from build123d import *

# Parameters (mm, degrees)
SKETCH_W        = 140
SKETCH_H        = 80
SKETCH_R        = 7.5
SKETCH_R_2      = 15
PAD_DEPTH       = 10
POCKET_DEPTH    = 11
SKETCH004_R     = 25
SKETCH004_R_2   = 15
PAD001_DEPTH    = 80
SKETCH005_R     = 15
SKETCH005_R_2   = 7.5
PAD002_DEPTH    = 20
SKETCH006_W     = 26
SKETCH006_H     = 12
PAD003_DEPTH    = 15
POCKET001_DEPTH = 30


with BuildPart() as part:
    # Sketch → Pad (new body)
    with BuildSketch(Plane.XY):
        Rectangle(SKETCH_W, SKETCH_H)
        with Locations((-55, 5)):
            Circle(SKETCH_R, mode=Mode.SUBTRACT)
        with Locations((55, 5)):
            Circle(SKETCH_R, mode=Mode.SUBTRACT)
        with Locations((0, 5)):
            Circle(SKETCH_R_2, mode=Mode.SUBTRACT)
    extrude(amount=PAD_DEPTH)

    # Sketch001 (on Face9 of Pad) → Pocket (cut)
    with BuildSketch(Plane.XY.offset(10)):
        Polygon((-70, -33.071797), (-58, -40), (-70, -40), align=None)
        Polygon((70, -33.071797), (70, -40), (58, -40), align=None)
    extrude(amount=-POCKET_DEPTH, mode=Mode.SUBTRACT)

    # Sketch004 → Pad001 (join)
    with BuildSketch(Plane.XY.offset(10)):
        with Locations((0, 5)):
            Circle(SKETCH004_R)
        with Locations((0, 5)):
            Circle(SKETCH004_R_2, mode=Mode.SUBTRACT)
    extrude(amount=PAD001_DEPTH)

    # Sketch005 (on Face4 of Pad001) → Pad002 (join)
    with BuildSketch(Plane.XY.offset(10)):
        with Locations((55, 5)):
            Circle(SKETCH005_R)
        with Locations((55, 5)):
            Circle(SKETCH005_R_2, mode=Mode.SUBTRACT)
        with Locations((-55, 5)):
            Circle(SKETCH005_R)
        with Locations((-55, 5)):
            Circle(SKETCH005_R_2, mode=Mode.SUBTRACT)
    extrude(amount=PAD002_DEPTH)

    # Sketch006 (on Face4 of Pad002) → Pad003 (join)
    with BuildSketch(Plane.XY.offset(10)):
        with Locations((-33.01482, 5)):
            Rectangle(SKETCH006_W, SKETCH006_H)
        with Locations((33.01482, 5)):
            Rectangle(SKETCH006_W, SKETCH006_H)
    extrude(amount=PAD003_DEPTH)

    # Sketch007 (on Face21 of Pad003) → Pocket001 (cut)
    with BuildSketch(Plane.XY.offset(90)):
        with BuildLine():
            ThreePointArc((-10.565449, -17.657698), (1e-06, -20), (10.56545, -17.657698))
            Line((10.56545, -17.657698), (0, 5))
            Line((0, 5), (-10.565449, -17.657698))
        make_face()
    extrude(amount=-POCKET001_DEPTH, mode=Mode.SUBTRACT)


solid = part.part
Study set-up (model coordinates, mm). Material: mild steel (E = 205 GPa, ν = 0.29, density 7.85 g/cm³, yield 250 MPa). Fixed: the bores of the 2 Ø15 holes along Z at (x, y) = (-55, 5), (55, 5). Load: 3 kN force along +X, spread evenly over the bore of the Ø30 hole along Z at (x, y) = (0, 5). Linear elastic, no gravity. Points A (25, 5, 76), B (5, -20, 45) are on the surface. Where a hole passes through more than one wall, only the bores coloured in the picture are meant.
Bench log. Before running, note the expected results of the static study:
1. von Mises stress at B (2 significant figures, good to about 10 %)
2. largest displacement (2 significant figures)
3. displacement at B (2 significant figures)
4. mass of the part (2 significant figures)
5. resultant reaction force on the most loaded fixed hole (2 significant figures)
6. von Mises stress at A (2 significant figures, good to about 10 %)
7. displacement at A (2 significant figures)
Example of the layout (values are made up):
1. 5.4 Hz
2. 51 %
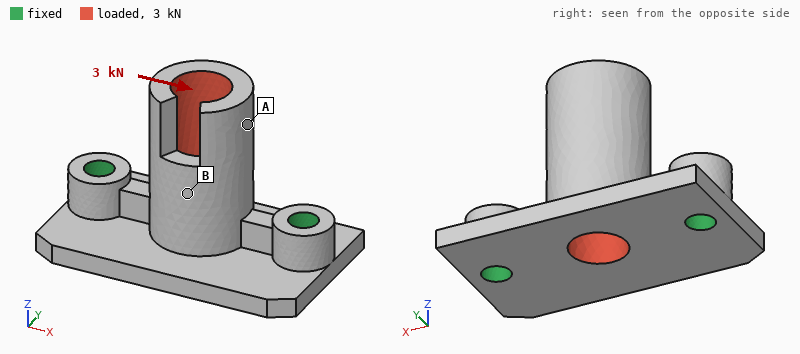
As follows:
1. 4.4 MPa
2. 9.0 µm
3. 3.2 µm
4. 1.7 kg
5. 2.0 kN
6. 1.9 MPa
7. 7.3 µm
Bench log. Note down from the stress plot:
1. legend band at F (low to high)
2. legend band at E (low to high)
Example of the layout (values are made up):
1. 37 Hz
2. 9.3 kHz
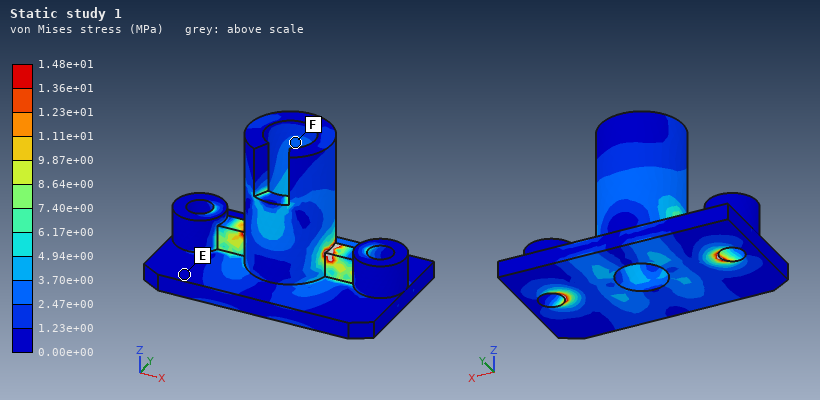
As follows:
1. 2.47e+00 to 3.70e+00 MPa
2. 0.00e+00 to 1.23e+00 MPa
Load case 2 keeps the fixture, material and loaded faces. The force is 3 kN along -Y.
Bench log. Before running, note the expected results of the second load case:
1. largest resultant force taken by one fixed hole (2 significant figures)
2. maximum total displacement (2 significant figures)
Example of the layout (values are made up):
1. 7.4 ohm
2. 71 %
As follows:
1. 1.5 kN
2. 42 µm
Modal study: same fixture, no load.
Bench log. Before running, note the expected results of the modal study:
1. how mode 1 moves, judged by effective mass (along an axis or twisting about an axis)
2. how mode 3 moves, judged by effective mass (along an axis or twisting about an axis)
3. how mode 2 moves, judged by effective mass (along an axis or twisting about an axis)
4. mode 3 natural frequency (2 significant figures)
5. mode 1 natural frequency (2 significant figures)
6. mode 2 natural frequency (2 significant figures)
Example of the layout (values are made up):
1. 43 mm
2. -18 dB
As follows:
1. along Y
2. along Z
3. along X
4. 5000 Hz
5. 1700 Hz
6. 3800 Hz
